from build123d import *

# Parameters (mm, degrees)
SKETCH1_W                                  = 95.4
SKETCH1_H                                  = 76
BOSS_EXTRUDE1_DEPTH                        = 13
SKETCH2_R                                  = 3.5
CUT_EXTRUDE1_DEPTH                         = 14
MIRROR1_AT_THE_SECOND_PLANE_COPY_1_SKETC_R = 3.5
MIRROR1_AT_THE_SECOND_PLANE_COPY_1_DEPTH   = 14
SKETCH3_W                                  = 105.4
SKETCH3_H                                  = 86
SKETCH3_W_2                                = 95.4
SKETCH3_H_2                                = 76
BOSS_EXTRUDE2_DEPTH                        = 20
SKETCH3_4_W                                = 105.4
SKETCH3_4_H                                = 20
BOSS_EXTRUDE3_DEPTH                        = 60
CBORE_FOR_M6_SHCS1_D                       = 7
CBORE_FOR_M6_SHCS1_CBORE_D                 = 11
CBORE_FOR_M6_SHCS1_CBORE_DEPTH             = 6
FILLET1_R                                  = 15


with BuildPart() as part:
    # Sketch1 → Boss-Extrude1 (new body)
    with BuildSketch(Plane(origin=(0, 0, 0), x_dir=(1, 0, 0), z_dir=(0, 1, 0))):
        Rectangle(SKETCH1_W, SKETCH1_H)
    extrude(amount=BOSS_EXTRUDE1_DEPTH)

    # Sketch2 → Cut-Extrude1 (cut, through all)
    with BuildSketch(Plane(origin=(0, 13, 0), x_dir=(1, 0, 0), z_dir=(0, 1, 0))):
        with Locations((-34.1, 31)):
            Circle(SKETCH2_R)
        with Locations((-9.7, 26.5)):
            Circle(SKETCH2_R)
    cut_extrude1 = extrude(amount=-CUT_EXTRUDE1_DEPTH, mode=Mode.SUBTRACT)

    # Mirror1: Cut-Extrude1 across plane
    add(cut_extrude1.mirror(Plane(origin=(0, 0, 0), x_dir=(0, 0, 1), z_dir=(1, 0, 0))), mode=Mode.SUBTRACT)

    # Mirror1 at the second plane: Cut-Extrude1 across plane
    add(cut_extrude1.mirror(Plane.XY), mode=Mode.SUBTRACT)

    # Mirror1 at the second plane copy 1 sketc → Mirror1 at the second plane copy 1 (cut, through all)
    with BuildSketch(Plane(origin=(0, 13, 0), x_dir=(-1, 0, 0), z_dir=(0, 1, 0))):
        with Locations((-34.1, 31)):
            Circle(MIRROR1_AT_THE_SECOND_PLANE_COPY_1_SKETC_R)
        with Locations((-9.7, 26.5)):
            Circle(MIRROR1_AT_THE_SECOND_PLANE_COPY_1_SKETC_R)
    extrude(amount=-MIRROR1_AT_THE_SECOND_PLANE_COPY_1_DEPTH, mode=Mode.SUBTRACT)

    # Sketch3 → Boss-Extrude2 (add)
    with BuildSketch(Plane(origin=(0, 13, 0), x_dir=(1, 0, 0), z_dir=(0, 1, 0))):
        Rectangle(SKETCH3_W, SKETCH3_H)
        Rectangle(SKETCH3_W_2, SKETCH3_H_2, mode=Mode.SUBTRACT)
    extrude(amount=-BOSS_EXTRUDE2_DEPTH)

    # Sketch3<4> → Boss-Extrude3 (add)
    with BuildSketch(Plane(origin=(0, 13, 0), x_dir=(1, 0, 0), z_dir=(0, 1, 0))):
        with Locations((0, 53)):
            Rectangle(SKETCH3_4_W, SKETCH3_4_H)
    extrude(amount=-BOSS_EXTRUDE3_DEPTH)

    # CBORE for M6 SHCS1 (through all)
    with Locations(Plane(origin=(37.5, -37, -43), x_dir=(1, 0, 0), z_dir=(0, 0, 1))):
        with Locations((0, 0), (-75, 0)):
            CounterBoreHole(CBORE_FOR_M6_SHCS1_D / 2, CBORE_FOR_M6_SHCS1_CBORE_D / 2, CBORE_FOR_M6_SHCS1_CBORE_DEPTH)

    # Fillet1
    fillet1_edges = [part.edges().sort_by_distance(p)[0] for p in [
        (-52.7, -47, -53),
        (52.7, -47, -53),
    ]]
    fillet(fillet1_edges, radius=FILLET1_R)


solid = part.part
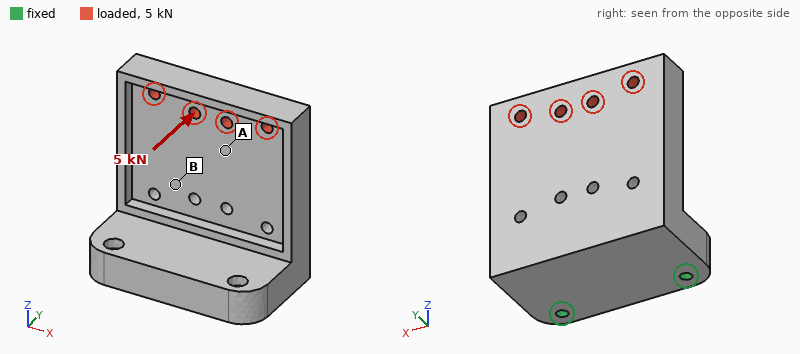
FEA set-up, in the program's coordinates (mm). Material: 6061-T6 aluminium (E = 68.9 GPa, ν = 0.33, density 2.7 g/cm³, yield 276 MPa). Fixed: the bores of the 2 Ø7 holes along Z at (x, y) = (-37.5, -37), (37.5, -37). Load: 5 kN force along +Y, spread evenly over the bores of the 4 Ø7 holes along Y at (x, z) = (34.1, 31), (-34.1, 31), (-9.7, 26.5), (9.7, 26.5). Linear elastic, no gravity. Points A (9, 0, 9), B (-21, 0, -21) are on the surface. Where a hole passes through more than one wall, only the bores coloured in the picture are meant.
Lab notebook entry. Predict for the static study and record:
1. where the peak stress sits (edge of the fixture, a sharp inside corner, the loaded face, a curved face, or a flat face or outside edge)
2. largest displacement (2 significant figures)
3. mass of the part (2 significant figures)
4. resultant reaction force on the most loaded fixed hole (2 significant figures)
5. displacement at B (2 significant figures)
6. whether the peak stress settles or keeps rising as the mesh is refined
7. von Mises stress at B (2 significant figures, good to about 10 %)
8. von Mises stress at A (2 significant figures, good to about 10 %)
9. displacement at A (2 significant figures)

edge of the fixture
1.1 mm
670 g
2.8 kN
0.29 mm
keeps rising
69 MPa
25 MPa
0.64 mm
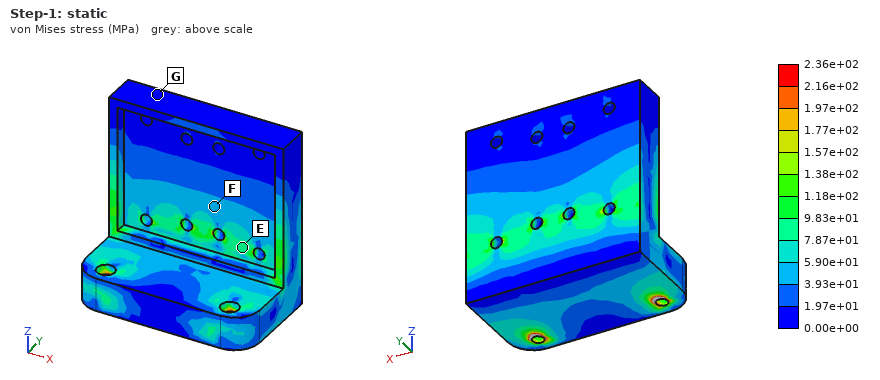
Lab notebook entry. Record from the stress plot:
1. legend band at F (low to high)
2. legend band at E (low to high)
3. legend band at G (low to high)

3.93e+01 to 5.90e+01 MPa
7.87e+01 to 9.83e+01 MPa
0.00e+00 to 1.97e+01 MPa
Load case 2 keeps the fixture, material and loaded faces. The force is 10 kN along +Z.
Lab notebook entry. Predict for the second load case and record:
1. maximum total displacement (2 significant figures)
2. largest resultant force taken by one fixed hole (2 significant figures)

0.51 mm
5.0 kN
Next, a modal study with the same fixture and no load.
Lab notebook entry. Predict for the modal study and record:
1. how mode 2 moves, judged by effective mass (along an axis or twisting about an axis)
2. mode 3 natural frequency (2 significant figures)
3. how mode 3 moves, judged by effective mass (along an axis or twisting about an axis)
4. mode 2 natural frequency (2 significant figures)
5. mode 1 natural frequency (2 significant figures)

along X
2600 Hz
along Z
1900 Hz
860 Hz
